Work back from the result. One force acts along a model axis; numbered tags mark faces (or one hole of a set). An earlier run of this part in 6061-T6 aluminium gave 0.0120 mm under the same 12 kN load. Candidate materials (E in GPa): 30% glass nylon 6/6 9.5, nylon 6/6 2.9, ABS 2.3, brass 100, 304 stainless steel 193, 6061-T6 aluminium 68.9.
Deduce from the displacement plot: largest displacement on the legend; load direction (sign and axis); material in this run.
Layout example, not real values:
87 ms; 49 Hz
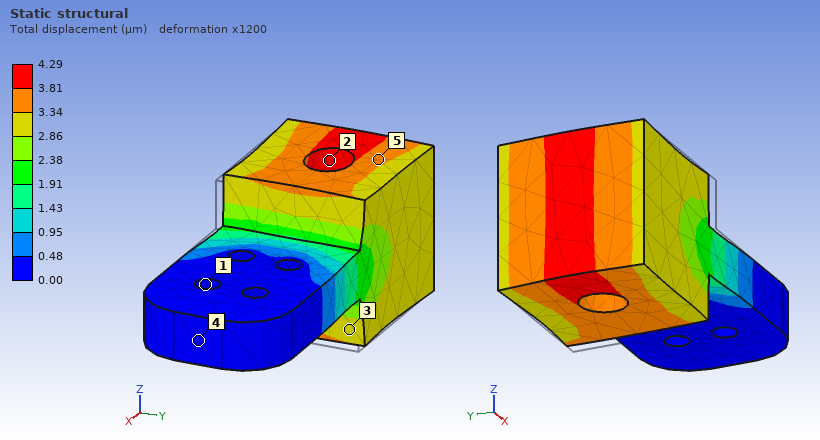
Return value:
4.29 µm; -X; 304 stainless steel
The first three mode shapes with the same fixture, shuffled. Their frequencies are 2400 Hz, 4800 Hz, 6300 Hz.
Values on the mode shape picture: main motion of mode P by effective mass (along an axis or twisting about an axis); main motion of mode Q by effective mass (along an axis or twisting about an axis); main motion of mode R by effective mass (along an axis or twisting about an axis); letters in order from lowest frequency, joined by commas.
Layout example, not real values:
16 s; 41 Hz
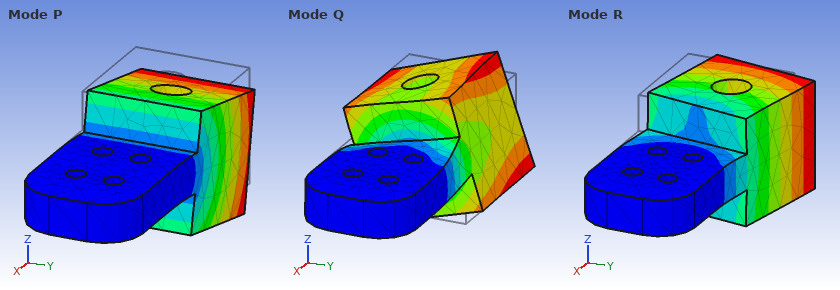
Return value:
along Z; twisting about X; along Y; P, R, Q
